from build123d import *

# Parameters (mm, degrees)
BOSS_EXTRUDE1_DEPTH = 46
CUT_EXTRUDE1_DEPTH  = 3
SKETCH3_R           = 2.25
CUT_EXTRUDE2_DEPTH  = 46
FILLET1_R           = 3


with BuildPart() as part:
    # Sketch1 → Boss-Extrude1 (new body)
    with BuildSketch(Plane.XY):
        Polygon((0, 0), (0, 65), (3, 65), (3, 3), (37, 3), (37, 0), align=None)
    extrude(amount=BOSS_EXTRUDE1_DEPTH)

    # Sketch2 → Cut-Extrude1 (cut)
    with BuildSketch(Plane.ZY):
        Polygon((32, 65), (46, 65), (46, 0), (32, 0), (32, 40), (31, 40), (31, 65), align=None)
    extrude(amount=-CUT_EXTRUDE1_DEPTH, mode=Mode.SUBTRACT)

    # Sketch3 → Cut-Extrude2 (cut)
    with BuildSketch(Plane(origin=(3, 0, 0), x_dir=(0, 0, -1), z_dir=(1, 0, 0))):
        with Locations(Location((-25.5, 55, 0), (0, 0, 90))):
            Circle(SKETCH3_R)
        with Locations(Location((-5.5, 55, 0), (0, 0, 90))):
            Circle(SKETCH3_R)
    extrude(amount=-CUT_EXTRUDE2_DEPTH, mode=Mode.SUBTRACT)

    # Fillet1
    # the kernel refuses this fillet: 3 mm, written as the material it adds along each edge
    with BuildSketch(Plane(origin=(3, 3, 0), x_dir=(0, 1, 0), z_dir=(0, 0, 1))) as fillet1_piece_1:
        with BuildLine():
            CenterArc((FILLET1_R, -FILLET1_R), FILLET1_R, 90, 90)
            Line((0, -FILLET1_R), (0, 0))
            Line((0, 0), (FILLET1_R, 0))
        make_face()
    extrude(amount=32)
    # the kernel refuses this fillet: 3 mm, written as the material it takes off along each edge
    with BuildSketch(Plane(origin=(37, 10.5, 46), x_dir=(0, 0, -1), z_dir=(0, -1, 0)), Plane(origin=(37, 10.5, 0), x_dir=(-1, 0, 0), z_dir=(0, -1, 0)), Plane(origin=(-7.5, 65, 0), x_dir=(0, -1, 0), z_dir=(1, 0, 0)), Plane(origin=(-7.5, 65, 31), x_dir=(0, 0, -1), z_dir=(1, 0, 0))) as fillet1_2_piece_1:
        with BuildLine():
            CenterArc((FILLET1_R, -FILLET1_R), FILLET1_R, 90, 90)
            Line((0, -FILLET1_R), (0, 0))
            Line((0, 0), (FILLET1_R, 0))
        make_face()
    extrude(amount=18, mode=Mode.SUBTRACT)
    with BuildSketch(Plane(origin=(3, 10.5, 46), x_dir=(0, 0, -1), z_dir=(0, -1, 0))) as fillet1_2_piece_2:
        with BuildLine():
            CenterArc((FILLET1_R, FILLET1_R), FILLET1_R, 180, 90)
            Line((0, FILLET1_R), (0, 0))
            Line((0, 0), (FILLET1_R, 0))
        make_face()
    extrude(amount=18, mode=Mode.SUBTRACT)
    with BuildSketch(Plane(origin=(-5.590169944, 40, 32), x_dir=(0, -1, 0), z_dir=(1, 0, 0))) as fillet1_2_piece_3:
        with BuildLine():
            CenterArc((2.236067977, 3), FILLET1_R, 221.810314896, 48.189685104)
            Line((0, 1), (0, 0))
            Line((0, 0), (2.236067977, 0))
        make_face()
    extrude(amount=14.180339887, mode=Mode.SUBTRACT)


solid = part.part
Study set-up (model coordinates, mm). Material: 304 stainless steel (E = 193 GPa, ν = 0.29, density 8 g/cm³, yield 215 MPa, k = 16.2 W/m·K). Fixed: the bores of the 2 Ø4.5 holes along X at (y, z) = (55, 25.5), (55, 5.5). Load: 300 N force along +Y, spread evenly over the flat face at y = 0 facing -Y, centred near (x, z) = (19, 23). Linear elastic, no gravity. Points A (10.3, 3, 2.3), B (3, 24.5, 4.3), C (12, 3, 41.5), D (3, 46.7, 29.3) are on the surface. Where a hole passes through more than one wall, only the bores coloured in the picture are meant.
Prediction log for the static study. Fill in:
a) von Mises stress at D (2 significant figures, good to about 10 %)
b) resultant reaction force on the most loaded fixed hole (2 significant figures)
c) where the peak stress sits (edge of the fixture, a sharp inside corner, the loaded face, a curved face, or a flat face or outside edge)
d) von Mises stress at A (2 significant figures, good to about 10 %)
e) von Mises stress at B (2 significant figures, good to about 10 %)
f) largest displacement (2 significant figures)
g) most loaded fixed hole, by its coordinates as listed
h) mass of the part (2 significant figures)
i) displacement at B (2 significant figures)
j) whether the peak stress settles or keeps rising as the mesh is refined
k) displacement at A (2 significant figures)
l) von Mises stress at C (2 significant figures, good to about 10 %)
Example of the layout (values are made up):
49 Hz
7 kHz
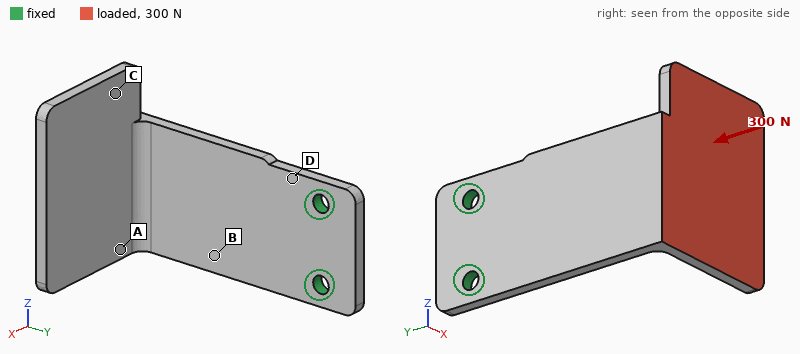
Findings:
130 MPa
250 N
edge of the fixture
50 MPa
110 MPa
0.96 mm
(55, 25.5)
86 g
0.16 mm
keeps rising
0.51 mm
15 MPa
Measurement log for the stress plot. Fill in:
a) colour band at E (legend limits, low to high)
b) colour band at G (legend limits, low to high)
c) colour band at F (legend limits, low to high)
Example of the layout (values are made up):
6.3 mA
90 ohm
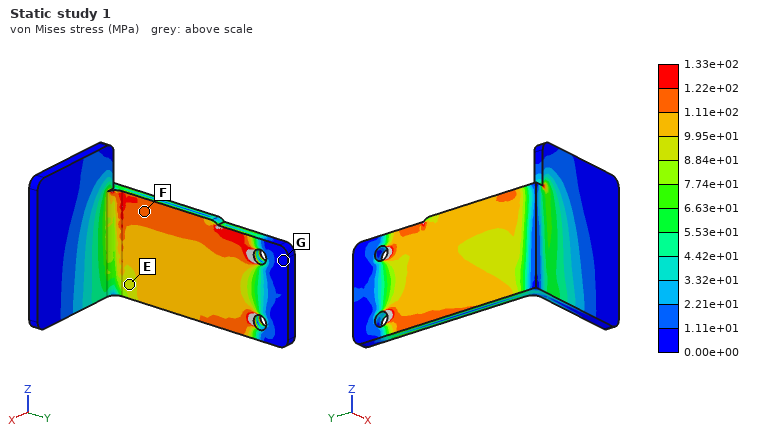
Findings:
8.84e+01 to 9.95e+01 MPa
0.00e+00 to 1.11e+01 MPa
1.11e+02 to 1.22e+02 MPa
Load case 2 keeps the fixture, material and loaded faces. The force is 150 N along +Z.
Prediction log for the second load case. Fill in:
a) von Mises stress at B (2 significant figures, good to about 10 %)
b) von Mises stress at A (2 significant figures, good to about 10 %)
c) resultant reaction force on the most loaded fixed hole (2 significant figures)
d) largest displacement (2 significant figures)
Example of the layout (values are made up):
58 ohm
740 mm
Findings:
49 MPa
16 MPa
400 N
0.23 mm
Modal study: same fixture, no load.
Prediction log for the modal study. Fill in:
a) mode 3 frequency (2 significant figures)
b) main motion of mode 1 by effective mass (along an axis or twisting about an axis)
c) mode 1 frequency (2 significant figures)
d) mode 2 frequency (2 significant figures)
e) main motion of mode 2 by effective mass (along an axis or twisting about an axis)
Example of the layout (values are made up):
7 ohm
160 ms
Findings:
1200 Hz
along X
340 Hz
720 Hz
along Z
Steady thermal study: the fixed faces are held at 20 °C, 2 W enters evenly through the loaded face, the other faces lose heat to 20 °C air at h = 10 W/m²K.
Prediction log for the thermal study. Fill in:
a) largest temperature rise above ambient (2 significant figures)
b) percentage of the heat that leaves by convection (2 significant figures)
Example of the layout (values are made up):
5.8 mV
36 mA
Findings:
41 K
63 %
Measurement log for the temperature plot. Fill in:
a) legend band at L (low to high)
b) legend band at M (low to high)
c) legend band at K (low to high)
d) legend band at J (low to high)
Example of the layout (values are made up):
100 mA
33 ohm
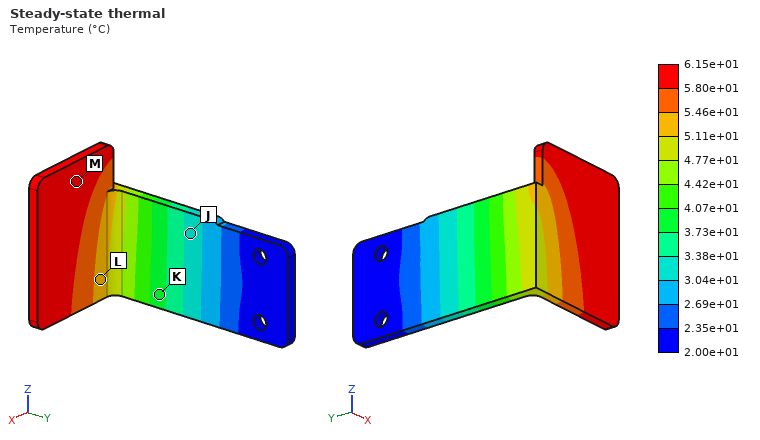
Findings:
5.11e+01 to 5.46e+01 °C
5.80e+01 to 6.15e+01 °C
3.73e+01 to 4.07e+01 °C
3.04e+01 to 3.38e+01 °C
